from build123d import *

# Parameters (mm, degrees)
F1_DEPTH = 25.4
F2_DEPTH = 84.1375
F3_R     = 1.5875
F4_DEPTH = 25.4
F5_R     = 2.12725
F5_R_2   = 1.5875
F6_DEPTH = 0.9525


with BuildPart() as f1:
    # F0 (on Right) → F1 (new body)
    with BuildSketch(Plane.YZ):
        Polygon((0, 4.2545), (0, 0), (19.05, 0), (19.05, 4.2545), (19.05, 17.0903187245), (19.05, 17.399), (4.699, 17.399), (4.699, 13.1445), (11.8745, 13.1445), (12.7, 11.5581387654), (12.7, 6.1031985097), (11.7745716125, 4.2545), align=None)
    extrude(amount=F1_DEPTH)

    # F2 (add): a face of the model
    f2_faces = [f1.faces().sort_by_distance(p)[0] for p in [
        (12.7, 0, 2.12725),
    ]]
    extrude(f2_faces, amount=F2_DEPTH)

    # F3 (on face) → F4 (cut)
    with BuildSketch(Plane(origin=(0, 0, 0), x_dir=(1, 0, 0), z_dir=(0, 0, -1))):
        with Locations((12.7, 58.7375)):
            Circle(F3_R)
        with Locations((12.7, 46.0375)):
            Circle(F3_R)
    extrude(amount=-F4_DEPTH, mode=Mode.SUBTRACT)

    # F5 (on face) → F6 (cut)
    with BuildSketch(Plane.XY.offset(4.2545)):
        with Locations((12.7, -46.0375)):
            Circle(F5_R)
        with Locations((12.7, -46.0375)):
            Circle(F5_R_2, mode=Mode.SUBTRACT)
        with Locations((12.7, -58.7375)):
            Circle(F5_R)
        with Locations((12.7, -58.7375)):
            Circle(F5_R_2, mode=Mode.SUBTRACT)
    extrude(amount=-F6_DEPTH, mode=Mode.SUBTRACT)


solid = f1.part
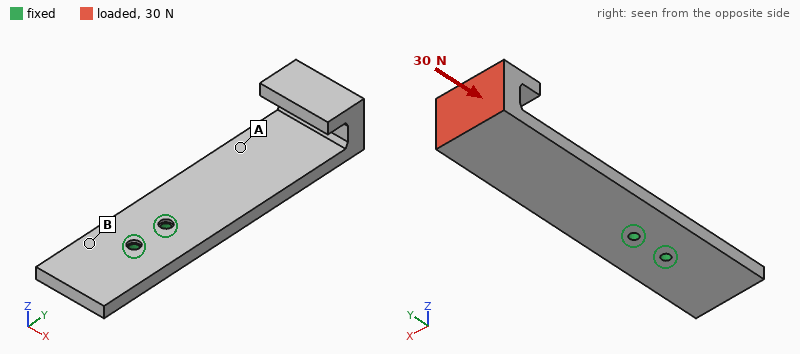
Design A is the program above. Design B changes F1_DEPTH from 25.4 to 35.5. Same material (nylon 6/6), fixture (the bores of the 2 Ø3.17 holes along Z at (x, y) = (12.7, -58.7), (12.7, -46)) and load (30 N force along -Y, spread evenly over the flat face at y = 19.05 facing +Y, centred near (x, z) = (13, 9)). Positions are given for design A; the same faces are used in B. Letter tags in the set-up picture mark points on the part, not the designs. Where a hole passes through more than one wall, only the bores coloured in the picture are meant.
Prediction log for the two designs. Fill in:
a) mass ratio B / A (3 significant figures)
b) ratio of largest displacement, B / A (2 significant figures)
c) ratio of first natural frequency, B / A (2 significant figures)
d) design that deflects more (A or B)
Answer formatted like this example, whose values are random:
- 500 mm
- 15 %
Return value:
- 1.40
- 0.74
- 0.97
- A
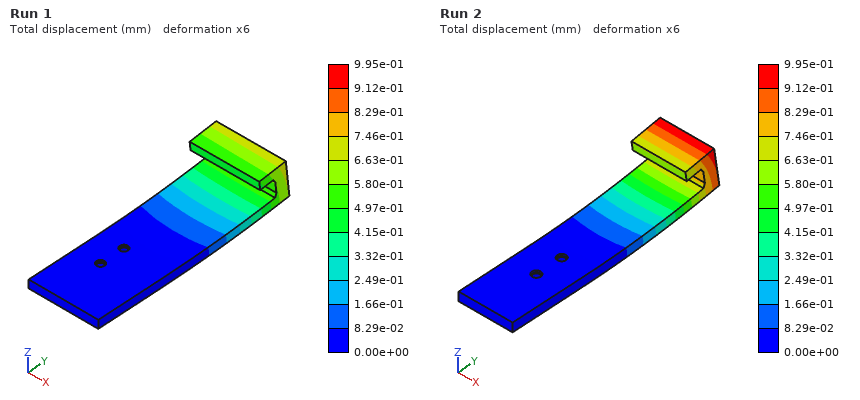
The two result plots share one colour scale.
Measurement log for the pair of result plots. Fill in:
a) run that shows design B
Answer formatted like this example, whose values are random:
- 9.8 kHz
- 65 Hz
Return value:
- Run 1
